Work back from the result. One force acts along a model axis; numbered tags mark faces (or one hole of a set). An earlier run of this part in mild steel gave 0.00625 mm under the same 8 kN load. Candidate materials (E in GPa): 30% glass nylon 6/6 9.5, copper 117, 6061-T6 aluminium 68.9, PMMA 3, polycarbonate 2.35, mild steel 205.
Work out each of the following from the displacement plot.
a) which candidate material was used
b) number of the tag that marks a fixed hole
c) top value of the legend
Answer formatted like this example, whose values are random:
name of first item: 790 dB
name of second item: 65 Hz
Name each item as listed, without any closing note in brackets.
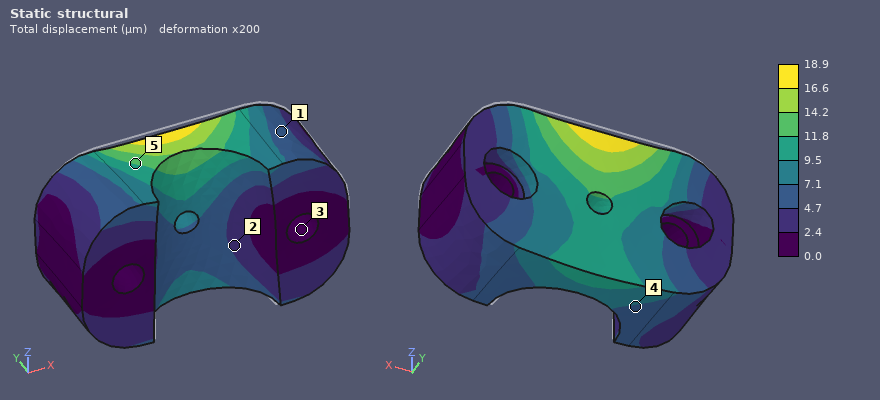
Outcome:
which candidate material was used: 6061-T6 aluminium
number of the tag that marks a fixed hole: 3
top value of the legend: 18.9 µm
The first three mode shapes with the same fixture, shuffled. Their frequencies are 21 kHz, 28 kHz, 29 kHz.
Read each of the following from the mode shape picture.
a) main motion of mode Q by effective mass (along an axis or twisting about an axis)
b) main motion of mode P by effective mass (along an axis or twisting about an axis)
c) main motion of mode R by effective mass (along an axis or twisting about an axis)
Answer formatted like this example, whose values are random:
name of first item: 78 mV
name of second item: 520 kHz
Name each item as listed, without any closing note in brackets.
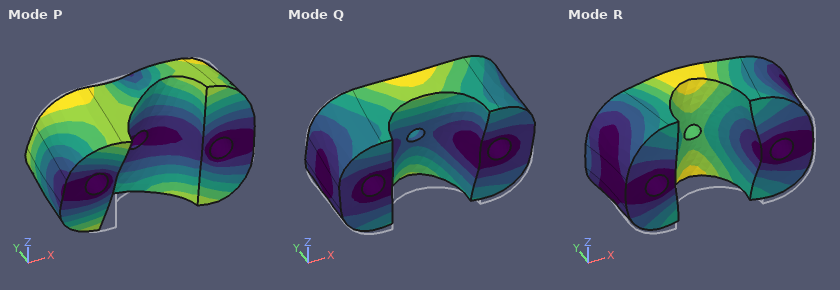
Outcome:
main motion of mode Q by effective mass: along Z
main motion of mode P by effective mass: twisting about Y
main motion of mode R by effective mass: along Y
